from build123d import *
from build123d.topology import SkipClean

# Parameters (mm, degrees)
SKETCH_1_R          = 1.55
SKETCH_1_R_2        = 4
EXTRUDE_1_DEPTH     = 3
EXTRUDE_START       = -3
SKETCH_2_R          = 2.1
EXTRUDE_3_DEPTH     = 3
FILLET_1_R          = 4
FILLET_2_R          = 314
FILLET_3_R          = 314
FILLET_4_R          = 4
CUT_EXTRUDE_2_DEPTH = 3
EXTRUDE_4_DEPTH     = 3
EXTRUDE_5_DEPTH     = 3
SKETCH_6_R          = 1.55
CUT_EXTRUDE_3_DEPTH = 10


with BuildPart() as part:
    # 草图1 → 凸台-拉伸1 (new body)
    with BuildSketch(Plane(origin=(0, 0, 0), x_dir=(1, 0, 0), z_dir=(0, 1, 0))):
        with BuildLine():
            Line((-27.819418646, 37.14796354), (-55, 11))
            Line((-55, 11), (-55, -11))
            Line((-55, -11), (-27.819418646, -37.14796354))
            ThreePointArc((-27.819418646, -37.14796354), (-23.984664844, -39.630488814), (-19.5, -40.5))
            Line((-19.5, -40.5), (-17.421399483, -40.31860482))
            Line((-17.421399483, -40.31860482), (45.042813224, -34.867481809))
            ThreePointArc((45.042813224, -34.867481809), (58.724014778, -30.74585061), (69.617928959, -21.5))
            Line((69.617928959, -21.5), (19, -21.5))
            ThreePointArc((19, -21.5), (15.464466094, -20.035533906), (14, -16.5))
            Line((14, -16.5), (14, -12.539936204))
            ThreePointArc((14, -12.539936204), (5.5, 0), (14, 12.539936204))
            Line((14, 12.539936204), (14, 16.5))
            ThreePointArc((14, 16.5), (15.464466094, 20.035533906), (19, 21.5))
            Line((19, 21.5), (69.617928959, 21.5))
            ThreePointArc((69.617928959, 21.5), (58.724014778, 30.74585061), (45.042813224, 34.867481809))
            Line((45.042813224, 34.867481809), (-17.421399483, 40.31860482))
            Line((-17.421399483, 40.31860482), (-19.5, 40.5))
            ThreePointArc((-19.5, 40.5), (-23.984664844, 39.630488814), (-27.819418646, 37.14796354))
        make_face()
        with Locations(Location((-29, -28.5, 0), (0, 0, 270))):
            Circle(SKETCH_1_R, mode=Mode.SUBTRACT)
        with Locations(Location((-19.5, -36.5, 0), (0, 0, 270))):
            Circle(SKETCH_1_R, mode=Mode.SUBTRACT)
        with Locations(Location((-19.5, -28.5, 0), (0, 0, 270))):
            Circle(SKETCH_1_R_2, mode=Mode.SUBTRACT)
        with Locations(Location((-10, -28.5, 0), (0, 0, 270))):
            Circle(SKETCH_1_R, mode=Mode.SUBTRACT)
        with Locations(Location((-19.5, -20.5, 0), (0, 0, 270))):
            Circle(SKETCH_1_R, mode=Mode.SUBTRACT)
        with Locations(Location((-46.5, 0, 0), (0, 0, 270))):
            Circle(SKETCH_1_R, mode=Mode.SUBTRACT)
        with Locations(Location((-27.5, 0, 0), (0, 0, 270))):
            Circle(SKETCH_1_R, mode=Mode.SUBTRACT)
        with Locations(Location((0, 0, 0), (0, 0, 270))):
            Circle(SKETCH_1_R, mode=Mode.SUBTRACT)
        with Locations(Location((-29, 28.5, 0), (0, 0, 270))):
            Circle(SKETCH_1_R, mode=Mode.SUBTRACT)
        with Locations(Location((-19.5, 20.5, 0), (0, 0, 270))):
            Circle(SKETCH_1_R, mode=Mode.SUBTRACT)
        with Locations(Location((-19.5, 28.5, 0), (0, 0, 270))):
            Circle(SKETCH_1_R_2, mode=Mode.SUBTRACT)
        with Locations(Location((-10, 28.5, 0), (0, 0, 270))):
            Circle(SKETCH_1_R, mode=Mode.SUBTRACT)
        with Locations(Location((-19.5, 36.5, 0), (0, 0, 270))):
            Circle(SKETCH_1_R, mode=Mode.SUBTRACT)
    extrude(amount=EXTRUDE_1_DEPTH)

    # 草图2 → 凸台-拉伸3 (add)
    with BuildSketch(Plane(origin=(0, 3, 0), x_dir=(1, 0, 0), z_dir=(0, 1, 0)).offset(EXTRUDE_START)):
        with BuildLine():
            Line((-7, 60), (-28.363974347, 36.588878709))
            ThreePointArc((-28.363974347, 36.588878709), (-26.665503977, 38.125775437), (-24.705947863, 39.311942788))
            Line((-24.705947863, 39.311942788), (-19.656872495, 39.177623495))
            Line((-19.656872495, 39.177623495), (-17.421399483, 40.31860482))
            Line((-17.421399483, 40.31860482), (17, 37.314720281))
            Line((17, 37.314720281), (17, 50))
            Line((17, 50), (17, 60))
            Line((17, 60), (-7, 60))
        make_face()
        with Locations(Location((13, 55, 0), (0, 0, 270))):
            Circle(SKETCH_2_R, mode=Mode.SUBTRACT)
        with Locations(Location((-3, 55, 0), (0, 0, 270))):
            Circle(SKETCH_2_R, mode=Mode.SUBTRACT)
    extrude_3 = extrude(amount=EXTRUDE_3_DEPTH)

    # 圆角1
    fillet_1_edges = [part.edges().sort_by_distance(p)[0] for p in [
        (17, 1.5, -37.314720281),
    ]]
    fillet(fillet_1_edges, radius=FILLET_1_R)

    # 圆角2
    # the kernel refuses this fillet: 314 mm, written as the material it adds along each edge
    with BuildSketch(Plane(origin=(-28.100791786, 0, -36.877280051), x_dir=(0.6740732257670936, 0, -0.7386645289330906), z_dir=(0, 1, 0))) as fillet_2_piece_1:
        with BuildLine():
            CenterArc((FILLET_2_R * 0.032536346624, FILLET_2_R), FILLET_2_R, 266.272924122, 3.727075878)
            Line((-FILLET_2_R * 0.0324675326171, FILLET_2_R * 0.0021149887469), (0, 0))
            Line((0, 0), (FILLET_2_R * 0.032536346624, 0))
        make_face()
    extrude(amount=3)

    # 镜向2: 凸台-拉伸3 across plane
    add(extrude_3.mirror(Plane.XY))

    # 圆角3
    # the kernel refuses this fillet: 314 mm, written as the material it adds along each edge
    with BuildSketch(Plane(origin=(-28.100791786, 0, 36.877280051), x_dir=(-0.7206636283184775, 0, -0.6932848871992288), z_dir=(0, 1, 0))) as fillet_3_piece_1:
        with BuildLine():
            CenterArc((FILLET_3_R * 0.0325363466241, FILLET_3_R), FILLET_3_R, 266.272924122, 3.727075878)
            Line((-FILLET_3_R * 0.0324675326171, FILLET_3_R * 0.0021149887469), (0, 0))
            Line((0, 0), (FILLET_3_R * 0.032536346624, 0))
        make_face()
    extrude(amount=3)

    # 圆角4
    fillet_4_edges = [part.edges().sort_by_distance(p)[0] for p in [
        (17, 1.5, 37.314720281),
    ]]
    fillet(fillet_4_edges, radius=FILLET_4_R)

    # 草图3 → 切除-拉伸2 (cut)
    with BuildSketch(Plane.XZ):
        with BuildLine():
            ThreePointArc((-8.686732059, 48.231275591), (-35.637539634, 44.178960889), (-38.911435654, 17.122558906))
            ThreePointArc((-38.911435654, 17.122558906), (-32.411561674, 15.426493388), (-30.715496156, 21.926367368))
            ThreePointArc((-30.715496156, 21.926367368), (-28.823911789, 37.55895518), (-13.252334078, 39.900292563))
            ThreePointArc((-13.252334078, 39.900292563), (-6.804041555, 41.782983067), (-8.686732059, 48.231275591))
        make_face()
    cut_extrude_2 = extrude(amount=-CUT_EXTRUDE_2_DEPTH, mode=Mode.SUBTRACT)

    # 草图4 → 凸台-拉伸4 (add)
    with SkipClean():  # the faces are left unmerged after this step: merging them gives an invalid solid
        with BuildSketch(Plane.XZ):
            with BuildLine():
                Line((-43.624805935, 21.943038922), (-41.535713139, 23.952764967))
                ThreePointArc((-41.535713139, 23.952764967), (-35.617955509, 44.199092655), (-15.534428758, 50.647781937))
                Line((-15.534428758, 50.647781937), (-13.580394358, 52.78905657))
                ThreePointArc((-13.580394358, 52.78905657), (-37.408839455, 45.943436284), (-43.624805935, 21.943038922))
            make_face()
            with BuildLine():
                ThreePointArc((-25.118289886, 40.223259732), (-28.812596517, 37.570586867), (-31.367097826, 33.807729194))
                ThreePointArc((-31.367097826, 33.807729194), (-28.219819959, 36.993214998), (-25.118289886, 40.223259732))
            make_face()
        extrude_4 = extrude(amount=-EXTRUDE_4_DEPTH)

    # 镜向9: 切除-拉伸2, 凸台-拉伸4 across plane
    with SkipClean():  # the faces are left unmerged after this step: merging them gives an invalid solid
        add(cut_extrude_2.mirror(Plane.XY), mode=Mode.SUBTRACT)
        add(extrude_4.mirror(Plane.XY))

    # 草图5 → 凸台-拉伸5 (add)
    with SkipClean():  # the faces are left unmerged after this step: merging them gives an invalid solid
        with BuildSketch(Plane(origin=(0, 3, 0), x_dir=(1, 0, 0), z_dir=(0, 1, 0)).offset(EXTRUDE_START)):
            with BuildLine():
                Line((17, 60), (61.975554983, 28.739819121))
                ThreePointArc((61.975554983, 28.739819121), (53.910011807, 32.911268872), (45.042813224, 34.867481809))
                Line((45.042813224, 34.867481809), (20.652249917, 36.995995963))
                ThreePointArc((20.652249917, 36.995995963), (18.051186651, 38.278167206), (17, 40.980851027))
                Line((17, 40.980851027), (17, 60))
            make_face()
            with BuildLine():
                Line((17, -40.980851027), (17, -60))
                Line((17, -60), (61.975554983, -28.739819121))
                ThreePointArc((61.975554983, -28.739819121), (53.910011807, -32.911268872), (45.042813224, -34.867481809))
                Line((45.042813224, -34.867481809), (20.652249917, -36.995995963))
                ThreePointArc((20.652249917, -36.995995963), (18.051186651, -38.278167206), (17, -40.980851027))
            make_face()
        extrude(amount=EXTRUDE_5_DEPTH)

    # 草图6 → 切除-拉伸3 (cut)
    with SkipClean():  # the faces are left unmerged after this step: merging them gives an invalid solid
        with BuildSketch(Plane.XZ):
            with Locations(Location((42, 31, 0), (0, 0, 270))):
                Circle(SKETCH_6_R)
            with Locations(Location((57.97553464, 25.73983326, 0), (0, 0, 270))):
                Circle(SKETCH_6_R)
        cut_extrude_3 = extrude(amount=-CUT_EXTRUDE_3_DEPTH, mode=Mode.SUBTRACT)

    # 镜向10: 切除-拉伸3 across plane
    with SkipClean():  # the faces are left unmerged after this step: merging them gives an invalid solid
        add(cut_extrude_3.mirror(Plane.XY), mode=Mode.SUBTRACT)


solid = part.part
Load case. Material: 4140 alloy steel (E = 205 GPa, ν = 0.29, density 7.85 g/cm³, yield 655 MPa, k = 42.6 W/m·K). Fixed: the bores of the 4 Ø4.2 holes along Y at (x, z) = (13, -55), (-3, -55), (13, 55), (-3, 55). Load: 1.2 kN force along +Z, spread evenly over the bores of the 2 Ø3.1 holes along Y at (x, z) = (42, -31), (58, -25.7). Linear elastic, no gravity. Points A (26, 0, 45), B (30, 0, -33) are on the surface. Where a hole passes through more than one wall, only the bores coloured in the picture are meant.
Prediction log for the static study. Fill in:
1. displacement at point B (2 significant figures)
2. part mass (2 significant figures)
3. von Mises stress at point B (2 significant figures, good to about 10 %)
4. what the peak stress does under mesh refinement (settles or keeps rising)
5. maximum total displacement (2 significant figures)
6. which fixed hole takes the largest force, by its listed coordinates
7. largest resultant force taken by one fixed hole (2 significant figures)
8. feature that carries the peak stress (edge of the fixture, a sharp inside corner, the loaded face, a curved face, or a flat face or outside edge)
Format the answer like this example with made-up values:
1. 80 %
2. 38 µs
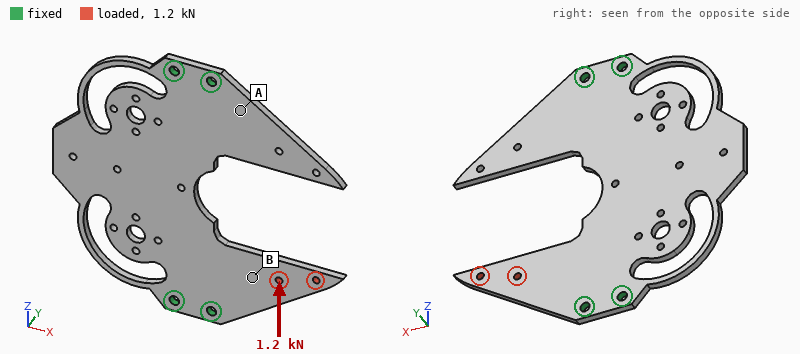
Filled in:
1. 13 µm
2. 180 g
3. 20 MPa
4. keeps rising
5. 60 µm
6. (13, -55)
7. 2.1 kN
8. edge of the fixture
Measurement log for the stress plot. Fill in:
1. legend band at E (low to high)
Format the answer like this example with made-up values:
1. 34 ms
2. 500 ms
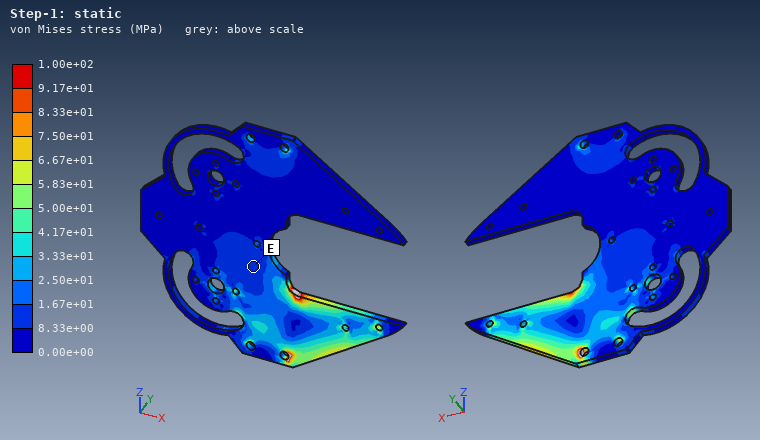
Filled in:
1. 8.33e+00 to 1.67e+01 MPa
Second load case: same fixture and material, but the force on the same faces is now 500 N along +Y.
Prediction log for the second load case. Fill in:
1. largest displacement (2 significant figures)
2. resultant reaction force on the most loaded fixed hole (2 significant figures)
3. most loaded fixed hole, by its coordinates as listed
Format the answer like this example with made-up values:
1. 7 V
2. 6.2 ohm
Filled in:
1. 1.9 mm
2. 990 N
3. (13, -55)
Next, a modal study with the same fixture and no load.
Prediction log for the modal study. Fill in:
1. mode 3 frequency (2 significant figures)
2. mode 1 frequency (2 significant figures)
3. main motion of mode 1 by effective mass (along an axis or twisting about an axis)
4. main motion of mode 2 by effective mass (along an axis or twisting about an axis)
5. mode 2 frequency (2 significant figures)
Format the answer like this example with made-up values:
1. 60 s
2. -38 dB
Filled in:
1. 1100 Hz
2. 640 Hz
3. along Y
4. along Y
5. 1000 Hz
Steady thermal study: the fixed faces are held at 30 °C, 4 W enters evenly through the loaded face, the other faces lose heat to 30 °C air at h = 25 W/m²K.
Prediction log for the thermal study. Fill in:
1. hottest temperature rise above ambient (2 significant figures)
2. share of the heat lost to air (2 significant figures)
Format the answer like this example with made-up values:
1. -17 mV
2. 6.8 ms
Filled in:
1. 49 K
2. 50 %
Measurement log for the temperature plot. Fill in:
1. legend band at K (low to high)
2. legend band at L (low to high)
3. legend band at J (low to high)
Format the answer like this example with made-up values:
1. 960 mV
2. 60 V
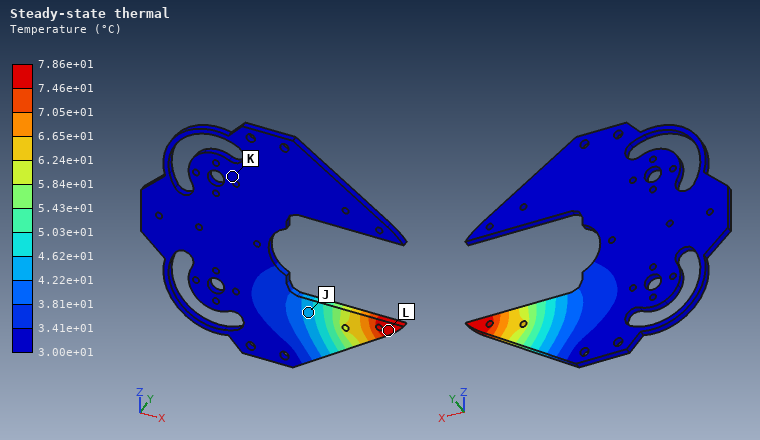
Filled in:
1. 3.00e+01 to 3.41e+01 °C
2. 7.46e+01 to 7.86e+01 °C
3. 4.22e+01 to 4.62e+01 °C
